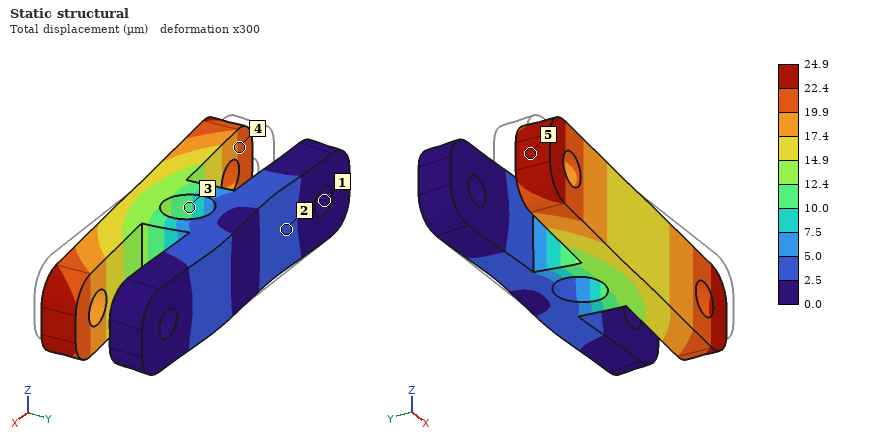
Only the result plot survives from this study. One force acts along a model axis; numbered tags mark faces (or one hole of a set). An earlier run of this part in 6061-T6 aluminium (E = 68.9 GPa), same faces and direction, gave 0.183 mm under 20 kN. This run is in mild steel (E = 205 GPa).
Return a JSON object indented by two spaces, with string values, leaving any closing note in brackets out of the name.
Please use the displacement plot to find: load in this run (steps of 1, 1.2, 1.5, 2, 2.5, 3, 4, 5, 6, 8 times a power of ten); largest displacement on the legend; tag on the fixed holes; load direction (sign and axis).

{
  "load in this run": "8 kN",
  "largest displacement on the legend": "24.9 µm",
  "tag on the fixed holes": "1",
  "load direction": "+X"
}
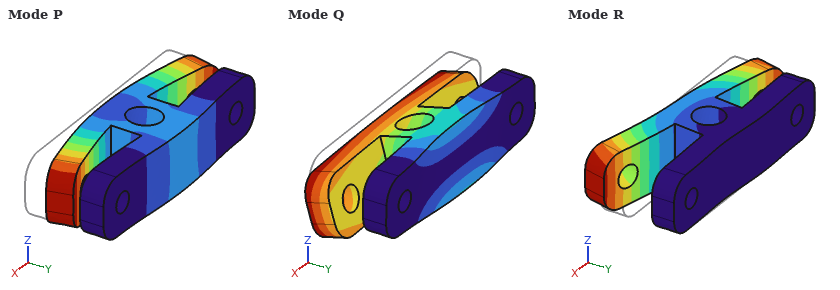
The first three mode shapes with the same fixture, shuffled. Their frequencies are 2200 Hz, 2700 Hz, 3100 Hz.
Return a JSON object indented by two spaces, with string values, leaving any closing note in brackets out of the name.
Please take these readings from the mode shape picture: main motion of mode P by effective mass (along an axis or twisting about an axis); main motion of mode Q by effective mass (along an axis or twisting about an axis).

{
  "main motion of mode P by effective mass": "along Y",
  "main motion of mode Q by effective mass": "along Z"
}
